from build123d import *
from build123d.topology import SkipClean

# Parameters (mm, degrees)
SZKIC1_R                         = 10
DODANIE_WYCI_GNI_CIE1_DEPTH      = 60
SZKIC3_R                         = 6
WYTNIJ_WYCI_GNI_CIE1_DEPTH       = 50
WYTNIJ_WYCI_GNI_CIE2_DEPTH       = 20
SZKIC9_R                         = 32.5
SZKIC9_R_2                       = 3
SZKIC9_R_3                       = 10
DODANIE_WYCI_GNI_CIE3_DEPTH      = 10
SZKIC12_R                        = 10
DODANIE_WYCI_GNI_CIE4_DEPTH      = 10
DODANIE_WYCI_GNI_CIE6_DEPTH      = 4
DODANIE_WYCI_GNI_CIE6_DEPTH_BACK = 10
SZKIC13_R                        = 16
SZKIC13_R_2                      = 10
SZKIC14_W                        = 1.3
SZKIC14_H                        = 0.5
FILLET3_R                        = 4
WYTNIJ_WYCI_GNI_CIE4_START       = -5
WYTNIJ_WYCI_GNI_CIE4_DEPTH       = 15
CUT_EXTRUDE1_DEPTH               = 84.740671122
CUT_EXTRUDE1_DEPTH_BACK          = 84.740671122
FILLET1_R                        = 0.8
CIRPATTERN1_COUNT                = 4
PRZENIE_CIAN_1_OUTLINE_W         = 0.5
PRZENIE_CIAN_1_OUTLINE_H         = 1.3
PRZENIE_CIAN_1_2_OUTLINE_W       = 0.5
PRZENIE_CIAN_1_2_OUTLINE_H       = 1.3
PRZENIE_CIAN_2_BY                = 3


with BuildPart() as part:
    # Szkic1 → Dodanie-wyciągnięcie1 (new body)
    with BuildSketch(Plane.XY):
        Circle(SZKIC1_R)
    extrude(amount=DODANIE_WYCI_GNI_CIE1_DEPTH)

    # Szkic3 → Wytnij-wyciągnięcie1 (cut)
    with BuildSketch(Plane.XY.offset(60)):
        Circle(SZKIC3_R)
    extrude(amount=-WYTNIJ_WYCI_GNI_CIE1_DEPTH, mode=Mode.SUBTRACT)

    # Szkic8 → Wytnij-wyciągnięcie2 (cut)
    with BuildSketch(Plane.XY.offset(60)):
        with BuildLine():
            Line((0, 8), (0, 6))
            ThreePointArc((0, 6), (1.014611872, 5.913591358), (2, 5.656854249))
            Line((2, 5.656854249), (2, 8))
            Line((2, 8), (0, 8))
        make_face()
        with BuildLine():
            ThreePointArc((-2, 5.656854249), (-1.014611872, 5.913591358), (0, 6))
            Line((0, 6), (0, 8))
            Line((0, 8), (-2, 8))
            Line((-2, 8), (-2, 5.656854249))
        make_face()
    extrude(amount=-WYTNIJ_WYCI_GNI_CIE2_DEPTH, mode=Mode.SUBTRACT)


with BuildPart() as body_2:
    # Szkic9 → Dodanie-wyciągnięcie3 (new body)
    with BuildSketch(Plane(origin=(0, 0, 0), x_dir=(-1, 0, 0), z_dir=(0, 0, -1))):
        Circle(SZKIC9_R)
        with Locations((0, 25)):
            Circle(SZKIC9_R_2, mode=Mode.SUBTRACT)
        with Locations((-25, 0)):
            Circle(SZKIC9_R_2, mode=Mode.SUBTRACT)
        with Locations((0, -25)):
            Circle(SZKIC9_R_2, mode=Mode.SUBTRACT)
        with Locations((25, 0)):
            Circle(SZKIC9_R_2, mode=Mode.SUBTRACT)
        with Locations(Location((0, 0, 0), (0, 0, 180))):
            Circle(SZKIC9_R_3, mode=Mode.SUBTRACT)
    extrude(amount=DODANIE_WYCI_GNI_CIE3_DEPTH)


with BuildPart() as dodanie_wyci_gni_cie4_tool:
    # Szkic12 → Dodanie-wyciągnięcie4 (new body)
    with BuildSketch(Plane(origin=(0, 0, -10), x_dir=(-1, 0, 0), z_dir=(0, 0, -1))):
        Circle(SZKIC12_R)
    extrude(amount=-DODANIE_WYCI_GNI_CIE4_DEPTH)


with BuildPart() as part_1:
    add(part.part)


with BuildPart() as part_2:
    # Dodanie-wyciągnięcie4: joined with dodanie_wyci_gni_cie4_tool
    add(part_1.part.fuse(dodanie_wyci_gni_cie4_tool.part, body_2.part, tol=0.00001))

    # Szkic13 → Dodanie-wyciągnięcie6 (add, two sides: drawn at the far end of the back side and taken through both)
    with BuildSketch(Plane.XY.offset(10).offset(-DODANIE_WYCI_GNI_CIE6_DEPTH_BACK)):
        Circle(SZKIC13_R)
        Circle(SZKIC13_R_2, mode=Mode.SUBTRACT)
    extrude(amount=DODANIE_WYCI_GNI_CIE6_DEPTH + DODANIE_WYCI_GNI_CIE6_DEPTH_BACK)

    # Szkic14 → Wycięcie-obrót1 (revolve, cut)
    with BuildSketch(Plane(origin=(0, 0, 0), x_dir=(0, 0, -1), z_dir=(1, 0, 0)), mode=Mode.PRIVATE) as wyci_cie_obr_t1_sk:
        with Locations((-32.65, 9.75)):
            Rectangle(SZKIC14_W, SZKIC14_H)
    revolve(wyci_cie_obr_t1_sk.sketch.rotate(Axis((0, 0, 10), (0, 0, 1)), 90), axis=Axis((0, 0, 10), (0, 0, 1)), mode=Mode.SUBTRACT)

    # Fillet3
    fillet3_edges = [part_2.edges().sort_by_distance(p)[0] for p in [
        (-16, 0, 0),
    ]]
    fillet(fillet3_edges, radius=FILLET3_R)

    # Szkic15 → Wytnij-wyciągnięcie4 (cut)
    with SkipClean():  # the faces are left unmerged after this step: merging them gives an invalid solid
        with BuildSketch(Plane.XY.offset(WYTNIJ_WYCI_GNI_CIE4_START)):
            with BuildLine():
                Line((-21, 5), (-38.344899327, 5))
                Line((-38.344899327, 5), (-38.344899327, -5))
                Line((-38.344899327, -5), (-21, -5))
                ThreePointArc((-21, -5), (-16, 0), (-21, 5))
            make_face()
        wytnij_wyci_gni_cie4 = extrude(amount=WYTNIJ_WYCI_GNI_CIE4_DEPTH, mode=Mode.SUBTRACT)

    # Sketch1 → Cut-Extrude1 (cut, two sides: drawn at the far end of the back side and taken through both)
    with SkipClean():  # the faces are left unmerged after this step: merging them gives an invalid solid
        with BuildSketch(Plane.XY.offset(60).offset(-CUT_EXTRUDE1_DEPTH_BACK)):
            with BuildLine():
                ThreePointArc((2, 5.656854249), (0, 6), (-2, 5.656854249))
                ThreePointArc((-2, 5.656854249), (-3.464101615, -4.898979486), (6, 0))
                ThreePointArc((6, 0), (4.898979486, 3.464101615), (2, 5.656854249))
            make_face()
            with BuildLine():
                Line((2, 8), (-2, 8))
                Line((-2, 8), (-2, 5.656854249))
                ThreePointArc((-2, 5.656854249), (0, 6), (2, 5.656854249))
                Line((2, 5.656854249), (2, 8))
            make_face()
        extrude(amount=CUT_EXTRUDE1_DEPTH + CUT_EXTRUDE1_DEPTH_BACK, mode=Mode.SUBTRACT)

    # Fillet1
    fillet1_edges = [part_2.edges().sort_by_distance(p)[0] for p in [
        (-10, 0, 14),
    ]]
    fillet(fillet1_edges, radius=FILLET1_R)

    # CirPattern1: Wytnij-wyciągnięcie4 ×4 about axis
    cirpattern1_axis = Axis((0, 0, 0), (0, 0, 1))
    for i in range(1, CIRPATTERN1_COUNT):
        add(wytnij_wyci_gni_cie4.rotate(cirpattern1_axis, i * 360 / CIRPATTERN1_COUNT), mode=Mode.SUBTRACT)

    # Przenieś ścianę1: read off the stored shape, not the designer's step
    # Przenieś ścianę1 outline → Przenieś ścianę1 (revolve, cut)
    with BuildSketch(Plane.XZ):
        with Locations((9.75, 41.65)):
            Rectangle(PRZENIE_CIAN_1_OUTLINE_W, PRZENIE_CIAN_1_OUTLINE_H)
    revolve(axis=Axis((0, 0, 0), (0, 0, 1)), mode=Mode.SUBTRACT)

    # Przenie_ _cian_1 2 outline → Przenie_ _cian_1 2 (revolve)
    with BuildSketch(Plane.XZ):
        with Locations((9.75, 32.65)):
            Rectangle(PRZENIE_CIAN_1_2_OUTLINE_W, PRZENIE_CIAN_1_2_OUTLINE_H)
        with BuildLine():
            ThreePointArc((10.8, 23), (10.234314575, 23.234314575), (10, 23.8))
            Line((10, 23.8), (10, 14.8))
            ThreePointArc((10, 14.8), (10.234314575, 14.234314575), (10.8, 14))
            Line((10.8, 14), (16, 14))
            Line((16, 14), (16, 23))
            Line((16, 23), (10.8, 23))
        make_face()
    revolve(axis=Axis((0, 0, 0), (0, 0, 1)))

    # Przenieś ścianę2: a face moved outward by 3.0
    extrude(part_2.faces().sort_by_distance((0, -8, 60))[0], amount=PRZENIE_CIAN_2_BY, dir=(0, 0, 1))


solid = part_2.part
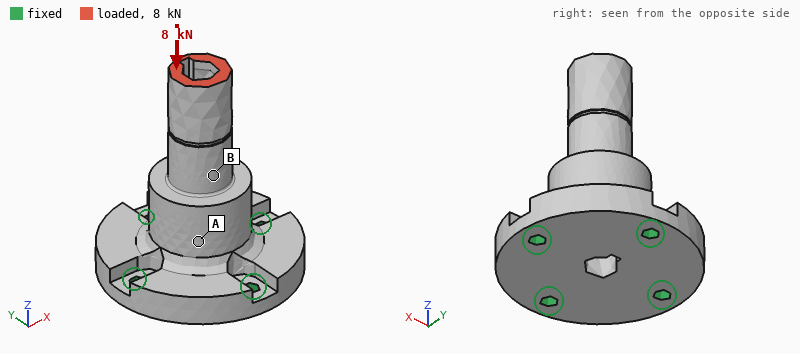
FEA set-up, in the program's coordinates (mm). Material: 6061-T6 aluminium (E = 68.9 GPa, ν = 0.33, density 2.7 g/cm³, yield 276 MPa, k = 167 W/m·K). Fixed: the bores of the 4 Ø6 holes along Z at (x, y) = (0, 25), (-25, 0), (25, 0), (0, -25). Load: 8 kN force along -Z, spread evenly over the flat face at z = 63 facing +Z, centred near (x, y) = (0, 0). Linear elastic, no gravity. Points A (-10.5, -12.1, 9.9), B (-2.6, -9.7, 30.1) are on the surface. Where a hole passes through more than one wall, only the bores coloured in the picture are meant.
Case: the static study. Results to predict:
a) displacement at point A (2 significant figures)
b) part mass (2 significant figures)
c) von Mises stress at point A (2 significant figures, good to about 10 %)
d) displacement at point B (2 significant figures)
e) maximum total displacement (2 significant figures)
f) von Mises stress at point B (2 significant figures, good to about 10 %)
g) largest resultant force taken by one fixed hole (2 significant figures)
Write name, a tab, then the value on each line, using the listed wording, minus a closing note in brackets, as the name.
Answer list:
displacement at point A	13 µm
part mass	140 g
von Mises stress at point A	11 MPa
displacement at point B	21 µm
maximum total displacement	42 µm
von Mises stress at point B	39 MPa
largest resultant force taken by one fixed hole	2.3 kN
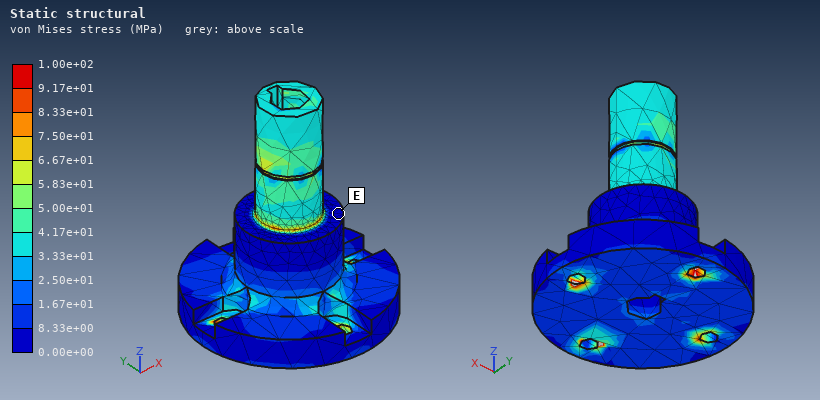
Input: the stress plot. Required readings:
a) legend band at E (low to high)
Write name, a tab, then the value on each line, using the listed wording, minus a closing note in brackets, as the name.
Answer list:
legend band at E	0.00e+00 to 8.33e+00 MPa
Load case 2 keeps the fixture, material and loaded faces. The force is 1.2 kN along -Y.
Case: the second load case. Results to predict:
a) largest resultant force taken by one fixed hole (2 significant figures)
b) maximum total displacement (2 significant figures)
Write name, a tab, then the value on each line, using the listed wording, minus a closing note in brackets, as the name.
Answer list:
largest resultant force taken by one fixed hole	1.9 kN
maximum total displacement	0.14 mm
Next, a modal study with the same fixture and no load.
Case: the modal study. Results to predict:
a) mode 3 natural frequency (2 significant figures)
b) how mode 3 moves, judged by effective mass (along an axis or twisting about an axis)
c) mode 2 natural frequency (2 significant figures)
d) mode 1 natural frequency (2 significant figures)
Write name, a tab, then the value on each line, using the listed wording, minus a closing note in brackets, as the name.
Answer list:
mode 3 natural frequency	13 kHz
how mode 3 moves, judged by effective mass	along Z
mode 2 natural frequency	5100 Hz
mode 1 natural frequency	5100 Hz
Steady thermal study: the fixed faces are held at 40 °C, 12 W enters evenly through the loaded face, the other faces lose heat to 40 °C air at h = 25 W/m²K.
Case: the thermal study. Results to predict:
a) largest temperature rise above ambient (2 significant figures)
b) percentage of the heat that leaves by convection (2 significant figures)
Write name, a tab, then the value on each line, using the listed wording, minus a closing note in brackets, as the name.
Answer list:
largest temperature rise above ambient	18 K
percentage of the heat that leaves by convection	13 %
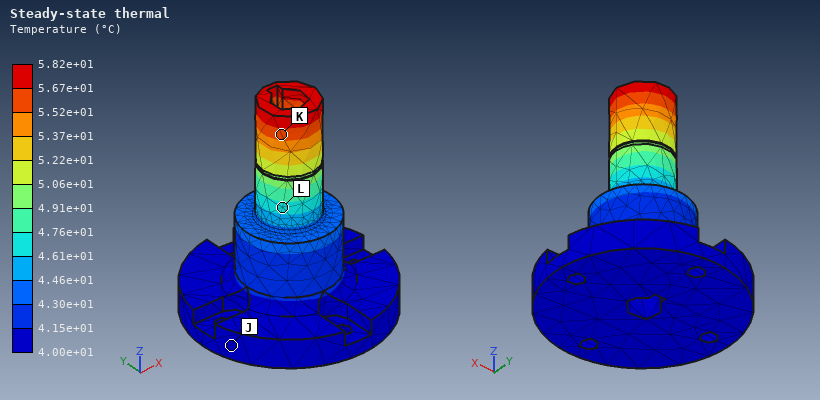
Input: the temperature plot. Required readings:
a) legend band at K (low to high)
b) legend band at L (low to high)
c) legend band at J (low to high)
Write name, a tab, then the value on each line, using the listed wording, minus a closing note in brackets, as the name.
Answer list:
legend band at K	5.52e+01 to 5.67e+01 °C
legend band at L	4.61e+01 to 4.76e+01 °C
legend band at J	4.00e+01 to 4.15e+01 °C
